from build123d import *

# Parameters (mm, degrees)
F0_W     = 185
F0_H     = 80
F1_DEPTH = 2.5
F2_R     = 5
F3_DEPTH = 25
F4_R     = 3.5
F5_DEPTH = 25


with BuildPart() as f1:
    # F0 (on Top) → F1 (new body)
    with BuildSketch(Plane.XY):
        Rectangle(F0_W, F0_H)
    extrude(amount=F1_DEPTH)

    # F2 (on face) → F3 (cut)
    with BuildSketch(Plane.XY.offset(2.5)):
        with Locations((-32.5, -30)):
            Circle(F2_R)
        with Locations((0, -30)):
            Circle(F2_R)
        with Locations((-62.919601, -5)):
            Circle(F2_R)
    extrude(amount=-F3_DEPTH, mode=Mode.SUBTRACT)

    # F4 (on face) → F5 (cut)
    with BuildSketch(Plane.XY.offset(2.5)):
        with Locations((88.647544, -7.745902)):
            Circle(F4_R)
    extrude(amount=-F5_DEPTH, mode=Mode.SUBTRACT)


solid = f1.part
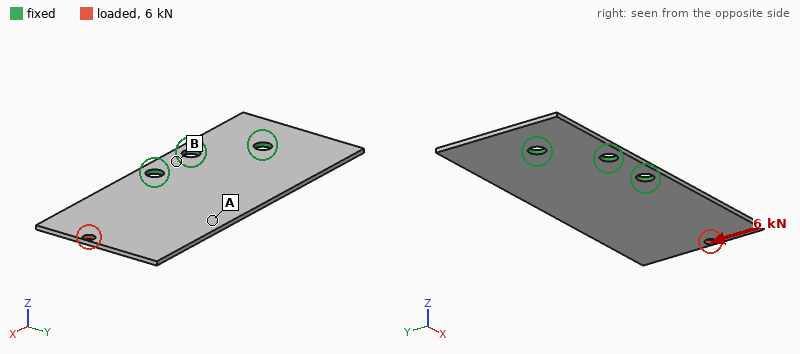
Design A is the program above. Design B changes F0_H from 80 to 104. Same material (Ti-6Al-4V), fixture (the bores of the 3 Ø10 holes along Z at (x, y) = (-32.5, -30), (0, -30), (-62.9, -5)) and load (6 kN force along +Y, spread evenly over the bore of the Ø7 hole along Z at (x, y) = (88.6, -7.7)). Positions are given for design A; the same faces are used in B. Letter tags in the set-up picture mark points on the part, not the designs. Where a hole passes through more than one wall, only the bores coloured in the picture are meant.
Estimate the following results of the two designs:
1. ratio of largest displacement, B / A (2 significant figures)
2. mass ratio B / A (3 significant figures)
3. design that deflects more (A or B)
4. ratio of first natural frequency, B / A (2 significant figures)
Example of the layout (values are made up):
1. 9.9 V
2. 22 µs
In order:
1. 0.71
2. 1.31
3. A
4. 0.95
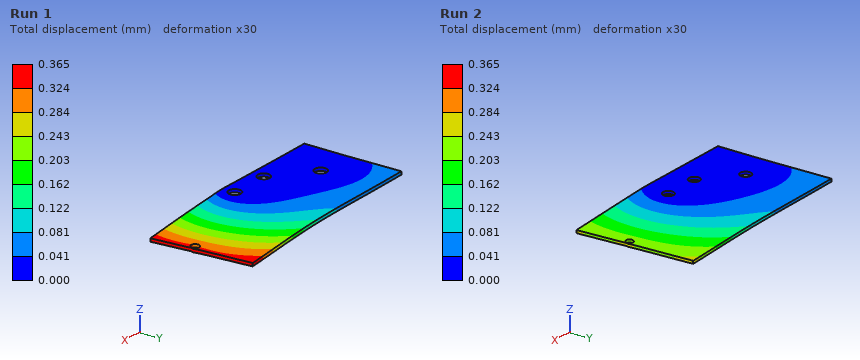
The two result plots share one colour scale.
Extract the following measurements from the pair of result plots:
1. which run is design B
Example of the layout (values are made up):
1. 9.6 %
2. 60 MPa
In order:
1. Run 2
